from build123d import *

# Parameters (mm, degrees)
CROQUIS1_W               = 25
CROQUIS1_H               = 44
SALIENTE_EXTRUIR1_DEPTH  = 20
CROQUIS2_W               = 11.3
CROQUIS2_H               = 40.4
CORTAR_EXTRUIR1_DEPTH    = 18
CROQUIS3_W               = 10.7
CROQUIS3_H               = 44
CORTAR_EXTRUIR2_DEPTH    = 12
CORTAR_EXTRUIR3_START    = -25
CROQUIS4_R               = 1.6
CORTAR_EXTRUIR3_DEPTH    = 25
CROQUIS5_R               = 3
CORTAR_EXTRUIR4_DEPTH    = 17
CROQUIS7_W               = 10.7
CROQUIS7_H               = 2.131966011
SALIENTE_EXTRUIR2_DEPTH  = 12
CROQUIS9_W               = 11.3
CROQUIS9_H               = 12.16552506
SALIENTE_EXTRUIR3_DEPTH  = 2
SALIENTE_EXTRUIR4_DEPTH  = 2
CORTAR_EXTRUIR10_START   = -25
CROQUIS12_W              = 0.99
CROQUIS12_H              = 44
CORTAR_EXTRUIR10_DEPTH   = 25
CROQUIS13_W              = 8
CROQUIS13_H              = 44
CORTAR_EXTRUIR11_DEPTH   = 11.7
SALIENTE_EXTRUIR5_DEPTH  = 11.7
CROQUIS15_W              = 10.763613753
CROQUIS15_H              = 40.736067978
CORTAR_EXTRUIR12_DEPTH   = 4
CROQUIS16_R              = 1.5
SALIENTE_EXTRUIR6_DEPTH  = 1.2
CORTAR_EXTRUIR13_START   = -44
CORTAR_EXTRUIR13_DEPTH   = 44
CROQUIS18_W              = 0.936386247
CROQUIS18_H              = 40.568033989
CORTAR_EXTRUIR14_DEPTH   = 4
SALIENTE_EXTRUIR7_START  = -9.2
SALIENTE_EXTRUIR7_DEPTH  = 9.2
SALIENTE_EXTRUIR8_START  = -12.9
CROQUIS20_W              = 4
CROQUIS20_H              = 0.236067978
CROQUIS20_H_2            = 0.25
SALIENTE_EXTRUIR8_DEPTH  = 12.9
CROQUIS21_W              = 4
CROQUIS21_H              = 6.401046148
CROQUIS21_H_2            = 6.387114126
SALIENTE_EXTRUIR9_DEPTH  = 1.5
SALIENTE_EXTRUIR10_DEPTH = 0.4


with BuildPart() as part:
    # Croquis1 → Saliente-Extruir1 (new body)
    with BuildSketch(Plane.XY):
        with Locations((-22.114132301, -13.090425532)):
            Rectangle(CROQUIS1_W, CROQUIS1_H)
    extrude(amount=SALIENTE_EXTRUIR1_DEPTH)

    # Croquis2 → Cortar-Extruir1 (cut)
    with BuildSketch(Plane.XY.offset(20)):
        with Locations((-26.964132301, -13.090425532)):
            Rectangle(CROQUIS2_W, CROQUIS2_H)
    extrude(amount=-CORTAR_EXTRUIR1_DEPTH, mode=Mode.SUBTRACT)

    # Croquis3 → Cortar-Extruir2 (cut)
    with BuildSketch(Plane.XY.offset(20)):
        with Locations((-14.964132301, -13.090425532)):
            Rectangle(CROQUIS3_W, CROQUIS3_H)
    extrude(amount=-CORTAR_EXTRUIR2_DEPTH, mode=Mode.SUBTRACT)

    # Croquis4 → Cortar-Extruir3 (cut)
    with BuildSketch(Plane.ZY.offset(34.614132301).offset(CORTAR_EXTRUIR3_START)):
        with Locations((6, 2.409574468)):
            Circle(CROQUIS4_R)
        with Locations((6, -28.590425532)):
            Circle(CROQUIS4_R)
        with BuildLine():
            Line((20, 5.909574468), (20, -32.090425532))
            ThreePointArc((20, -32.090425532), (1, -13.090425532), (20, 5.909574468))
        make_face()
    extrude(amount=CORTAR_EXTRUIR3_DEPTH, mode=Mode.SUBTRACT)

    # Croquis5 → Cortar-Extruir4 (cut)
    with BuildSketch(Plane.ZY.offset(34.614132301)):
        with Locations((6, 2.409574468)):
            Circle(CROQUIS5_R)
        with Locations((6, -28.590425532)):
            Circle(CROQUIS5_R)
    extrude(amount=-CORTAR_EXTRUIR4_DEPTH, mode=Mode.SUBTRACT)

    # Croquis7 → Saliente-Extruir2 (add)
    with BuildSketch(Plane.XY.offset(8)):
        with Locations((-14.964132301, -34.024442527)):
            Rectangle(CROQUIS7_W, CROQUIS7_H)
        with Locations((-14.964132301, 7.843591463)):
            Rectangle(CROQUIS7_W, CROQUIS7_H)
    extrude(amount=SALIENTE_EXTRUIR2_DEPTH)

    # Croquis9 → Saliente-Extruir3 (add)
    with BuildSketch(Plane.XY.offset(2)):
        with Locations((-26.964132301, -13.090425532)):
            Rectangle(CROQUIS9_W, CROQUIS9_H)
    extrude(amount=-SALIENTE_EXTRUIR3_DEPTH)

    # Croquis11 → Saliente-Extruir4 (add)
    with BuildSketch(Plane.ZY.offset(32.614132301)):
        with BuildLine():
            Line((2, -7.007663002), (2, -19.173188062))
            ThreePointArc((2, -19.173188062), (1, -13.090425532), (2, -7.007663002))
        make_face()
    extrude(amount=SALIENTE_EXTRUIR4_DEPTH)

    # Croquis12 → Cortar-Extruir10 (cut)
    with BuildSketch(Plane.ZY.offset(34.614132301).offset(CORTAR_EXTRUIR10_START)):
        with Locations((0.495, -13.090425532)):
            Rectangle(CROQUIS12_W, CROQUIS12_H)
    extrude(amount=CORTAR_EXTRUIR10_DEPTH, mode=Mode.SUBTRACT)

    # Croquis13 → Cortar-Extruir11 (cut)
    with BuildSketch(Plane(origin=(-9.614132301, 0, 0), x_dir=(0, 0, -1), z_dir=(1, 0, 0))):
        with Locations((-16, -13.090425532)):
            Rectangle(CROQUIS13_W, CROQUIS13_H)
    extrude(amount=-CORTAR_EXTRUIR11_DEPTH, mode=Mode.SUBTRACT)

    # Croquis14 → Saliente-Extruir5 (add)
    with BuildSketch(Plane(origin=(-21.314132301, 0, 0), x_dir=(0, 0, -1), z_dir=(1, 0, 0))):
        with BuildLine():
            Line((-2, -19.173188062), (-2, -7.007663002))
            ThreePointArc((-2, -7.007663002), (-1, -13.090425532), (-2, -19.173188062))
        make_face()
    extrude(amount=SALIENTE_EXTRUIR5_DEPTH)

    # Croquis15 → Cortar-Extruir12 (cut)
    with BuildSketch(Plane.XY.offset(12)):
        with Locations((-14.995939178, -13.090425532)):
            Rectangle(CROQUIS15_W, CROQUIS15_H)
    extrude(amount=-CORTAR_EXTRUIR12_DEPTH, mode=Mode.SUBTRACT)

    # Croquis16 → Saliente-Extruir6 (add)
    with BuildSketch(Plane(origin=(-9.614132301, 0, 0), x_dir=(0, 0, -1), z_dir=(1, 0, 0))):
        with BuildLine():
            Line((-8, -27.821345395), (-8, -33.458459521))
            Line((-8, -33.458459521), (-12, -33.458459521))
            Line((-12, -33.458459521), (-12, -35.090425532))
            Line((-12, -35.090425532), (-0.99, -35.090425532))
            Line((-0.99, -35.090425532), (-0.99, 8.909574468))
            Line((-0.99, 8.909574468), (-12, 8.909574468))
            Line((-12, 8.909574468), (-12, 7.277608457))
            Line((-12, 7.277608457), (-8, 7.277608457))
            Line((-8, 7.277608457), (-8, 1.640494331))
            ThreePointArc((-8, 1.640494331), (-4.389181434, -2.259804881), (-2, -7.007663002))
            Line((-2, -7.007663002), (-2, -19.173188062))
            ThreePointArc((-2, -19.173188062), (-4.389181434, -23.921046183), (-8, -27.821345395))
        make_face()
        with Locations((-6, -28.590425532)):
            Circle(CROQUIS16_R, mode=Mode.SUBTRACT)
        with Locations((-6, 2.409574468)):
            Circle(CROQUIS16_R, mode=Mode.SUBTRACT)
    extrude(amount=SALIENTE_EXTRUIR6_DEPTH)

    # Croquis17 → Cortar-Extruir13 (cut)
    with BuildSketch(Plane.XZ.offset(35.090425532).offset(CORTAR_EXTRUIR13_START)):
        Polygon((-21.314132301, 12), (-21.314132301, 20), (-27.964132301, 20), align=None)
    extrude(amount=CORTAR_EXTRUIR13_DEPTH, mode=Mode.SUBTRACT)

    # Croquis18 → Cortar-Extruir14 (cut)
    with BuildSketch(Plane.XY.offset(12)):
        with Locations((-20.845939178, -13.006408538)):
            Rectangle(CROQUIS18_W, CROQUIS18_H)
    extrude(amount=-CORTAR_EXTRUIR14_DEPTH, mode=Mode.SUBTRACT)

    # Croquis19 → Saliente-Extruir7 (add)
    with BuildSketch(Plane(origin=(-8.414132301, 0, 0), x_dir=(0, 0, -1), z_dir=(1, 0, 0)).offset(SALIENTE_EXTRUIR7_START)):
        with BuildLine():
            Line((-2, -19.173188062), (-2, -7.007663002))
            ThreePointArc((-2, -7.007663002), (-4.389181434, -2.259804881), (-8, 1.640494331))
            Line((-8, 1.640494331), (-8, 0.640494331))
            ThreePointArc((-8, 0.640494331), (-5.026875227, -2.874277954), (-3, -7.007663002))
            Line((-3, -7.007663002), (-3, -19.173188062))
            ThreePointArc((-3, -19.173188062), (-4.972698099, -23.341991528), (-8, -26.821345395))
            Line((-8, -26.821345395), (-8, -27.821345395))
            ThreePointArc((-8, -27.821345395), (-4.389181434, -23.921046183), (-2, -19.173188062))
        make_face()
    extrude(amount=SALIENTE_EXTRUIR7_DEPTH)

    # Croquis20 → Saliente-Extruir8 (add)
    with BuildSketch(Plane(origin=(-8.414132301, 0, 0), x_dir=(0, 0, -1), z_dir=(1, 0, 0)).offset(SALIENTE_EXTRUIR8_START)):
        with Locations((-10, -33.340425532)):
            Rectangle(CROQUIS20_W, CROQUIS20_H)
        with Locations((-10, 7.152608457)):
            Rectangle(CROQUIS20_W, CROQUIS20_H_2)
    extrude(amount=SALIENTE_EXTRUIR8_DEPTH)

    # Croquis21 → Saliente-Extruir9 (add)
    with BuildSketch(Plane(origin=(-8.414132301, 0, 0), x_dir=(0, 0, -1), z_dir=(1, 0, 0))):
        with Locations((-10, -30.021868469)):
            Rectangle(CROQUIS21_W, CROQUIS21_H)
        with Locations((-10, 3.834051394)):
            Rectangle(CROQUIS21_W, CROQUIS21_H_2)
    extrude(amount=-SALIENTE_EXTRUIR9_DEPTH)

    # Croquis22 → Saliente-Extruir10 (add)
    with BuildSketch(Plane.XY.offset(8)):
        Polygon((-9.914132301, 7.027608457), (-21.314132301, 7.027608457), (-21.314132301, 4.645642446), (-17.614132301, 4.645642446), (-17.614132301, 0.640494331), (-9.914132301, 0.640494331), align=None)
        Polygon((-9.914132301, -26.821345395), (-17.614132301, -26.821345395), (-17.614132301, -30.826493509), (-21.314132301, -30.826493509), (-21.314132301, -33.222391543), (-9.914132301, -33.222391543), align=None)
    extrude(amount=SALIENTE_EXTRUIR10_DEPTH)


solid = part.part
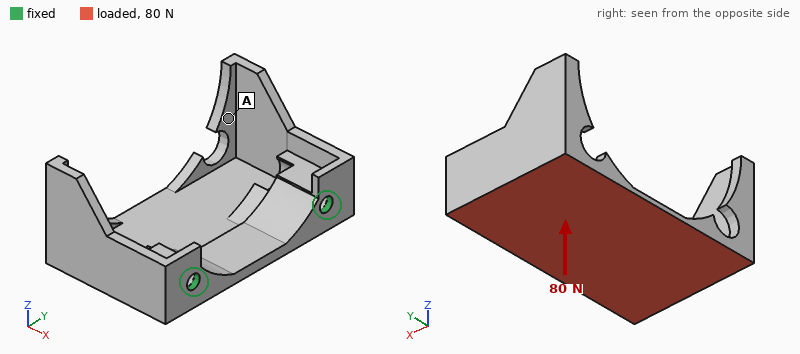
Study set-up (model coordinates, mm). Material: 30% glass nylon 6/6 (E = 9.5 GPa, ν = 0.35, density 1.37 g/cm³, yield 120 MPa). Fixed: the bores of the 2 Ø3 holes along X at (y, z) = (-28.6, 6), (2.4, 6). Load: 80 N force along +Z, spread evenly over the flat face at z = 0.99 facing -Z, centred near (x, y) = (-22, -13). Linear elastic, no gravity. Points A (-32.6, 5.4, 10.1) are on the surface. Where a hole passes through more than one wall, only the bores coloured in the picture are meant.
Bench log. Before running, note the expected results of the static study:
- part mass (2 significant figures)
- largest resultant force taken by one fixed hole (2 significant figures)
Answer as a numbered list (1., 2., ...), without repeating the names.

1. 5.6 g
2. 43 N
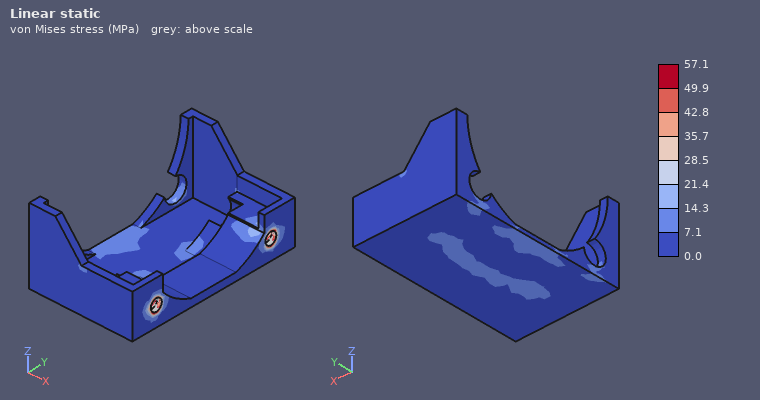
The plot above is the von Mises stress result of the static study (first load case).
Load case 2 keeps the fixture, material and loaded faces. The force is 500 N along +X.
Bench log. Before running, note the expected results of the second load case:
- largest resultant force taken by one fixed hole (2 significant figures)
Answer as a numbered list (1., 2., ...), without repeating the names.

1. 250 N
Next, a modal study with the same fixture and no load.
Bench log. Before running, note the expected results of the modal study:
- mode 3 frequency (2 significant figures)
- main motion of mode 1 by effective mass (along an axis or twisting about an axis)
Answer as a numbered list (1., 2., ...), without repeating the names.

1. 2500 Hz
2. along Z
